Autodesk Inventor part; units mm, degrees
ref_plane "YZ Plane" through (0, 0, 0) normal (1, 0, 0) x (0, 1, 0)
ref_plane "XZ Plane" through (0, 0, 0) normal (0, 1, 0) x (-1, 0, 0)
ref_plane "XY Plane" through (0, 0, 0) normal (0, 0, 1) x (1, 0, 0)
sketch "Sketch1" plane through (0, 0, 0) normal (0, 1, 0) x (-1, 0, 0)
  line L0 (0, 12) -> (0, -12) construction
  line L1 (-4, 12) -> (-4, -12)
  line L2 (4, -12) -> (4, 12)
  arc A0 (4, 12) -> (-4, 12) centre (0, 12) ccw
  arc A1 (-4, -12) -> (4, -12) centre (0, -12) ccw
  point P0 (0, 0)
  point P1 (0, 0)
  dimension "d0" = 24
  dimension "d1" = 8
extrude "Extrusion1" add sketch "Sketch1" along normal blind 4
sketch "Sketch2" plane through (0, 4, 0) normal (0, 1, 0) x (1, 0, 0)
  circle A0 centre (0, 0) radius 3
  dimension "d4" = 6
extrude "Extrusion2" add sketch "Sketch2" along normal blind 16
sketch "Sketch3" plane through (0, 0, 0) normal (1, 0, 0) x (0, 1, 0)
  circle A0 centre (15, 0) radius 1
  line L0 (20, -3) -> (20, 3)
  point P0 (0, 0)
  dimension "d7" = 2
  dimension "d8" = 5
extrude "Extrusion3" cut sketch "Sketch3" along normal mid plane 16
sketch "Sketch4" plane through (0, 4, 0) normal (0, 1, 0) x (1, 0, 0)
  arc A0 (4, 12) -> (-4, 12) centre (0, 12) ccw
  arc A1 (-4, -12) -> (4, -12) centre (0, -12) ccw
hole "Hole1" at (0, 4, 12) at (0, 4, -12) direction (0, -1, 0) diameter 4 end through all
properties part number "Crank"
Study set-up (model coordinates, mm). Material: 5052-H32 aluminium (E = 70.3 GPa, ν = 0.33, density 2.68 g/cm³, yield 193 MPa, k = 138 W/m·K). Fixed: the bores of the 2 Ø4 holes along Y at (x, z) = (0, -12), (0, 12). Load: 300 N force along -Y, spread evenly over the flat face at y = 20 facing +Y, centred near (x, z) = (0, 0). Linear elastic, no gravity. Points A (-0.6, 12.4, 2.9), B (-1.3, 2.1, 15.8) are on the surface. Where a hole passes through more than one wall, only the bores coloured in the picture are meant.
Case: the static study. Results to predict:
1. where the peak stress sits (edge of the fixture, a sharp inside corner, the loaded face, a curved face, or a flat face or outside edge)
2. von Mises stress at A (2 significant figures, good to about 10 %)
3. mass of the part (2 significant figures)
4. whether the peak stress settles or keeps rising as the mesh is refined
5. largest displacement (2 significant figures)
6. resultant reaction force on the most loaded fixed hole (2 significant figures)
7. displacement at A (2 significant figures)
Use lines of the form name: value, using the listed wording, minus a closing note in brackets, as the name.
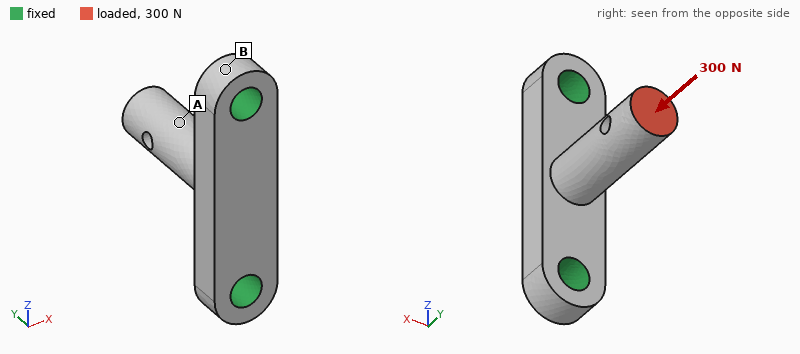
where the peak stress sits: edge of the fixture
von Mises stress at A: 15 MPa
mass of the part: 3.5 g
whether the peak stress settles or keeps rising as the mesh is refined: keeps rising
largest displacement: 8.3 µm
resultant reaction force on the most loaded fixed hole: 150 N
displacement at A: 6.8 µm
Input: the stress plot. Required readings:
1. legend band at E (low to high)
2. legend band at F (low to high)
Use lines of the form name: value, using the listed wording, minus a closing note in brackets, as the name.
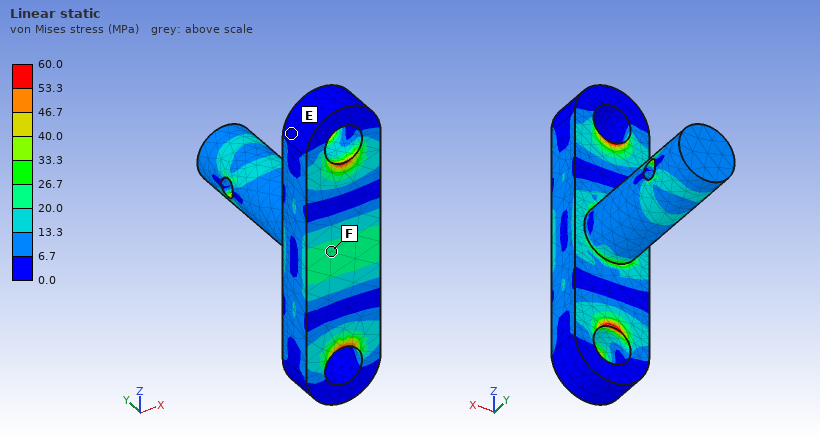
legend band at E: 0.0 to 6.7 MPa
legend band at F: 20.0 to 26.7 MPa
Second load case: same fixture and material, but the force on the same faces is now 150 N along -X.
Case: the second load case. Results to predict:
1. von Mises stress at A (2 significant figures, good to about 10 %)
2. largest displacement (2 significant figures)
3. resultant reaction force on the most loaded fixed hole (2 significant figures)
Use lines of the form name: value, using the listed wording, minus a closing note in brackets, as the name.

von Mises stress at A: 15 MPa
largest displacement: 0.13 mm
resultant reaction force on the most loaded fixed hole: 75 N
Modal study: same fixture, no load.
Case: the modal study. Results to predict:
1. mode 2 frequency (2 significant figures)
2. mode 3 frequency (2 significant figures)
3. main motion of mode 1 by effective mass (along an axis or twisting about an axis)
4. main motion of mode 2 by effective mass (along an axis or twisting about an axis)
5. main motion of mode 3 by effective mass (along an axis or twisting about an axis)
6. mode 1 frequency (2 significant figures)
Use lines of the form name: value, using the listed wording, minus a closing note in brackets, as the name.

mode 2 frequency: 12 kHz
mode 3 frequency: 26 kHz
main motion of mode 1 by effective mass: along X
main motion of mode 2 by effective mass: along Z
main motion of mode 3 by effective mass: along Y
mode 1 frequency: 8900 Hz
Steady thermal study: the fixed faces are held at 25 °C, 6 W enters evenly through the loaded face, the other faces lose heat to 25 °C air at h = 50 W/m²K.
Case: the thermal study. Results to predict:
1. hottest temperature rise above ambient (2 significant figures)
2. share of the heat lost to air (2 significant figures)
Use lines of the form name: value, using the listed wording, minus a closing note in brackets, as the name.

hottest temperature rise above ambient: 33 K
share of the heat lost to air: 6.8 %
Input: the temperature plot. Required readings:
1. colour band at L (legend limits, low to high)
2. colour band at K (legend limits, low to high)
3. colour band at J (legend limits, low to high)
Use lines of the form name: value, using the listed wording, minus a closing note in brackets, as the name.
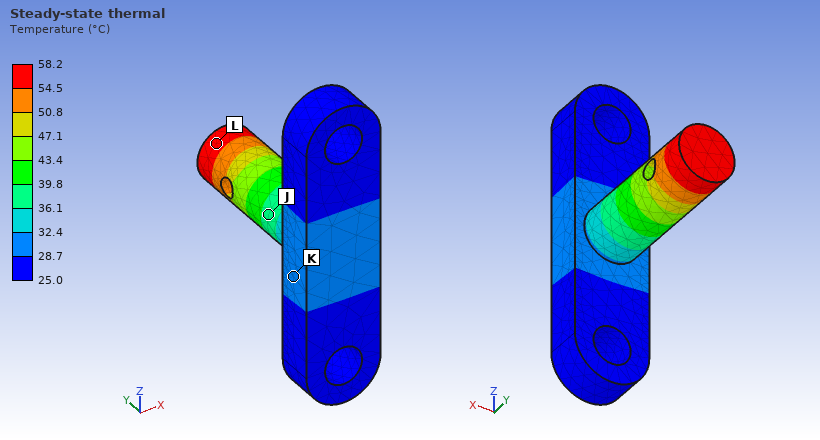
colour band at L: 54.5 to 58.2 °C
colour band at K: 28.7 to 32.4 °C
colour band at J: 36.1 to 39.8 °C
